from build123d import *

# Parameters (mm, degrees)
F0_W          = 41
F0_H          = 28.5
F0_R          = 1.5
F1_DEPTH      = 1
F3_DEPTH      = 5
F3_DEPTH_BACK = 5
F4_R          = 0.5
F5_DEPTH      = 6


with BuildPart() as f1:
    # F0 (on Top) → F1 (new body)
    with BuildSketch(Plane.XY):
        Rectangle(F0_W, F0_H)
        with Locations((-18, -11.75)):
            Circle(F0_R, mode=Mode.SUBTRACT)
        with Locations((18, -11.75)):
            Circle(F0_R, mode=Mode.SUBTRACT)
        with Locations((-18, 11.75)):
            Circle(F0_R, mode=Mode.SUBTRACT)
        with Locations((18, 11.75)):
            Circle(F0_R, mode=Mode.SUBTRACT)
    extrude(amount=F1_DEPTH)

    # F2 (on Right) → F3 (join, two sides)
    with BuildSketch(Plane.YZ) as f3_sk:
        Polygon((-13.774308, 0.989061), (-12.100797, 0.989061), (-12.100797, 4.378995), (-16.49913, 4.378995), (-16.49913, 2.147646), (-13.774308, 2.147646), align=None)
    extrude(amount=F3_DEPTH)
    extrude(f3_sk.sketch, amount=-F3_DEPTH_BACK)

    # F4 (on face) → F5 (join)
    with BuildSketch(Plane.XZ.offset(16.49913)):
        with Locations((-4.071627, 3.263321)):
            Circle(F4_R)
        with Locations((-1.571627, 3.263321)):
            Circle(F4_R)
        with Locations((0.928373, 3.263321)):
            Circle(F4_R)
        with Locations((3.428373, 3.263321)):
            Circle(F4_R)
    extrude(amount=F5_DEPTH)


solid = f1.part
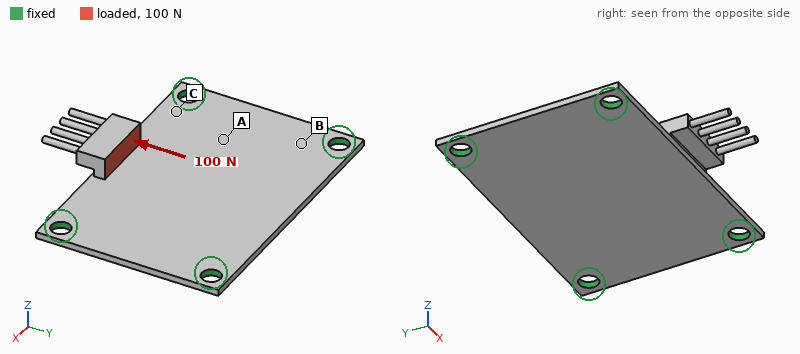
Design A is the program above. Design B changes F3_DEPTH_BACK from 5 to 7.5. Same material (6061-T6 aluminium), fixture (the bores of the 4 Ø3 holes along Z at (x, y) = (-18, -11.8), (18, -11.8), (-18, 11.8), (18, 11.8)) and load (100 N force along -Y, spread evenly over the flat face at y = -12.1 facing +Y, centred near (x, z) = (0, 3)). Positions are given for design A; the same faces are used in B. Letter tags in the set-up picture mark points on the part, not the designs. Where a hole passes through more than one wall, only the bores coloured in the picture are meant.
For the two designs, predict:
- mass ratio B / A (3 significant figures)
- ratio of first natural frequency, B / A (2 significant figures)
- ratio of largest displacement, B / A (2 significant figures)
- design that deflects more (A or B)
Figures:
1.02
1.0
0.86
A
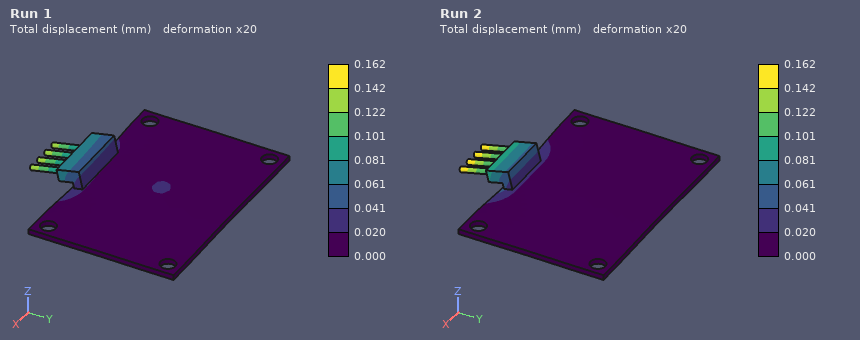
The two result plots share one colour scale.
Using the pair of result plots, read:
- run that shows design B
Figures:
Run 1
